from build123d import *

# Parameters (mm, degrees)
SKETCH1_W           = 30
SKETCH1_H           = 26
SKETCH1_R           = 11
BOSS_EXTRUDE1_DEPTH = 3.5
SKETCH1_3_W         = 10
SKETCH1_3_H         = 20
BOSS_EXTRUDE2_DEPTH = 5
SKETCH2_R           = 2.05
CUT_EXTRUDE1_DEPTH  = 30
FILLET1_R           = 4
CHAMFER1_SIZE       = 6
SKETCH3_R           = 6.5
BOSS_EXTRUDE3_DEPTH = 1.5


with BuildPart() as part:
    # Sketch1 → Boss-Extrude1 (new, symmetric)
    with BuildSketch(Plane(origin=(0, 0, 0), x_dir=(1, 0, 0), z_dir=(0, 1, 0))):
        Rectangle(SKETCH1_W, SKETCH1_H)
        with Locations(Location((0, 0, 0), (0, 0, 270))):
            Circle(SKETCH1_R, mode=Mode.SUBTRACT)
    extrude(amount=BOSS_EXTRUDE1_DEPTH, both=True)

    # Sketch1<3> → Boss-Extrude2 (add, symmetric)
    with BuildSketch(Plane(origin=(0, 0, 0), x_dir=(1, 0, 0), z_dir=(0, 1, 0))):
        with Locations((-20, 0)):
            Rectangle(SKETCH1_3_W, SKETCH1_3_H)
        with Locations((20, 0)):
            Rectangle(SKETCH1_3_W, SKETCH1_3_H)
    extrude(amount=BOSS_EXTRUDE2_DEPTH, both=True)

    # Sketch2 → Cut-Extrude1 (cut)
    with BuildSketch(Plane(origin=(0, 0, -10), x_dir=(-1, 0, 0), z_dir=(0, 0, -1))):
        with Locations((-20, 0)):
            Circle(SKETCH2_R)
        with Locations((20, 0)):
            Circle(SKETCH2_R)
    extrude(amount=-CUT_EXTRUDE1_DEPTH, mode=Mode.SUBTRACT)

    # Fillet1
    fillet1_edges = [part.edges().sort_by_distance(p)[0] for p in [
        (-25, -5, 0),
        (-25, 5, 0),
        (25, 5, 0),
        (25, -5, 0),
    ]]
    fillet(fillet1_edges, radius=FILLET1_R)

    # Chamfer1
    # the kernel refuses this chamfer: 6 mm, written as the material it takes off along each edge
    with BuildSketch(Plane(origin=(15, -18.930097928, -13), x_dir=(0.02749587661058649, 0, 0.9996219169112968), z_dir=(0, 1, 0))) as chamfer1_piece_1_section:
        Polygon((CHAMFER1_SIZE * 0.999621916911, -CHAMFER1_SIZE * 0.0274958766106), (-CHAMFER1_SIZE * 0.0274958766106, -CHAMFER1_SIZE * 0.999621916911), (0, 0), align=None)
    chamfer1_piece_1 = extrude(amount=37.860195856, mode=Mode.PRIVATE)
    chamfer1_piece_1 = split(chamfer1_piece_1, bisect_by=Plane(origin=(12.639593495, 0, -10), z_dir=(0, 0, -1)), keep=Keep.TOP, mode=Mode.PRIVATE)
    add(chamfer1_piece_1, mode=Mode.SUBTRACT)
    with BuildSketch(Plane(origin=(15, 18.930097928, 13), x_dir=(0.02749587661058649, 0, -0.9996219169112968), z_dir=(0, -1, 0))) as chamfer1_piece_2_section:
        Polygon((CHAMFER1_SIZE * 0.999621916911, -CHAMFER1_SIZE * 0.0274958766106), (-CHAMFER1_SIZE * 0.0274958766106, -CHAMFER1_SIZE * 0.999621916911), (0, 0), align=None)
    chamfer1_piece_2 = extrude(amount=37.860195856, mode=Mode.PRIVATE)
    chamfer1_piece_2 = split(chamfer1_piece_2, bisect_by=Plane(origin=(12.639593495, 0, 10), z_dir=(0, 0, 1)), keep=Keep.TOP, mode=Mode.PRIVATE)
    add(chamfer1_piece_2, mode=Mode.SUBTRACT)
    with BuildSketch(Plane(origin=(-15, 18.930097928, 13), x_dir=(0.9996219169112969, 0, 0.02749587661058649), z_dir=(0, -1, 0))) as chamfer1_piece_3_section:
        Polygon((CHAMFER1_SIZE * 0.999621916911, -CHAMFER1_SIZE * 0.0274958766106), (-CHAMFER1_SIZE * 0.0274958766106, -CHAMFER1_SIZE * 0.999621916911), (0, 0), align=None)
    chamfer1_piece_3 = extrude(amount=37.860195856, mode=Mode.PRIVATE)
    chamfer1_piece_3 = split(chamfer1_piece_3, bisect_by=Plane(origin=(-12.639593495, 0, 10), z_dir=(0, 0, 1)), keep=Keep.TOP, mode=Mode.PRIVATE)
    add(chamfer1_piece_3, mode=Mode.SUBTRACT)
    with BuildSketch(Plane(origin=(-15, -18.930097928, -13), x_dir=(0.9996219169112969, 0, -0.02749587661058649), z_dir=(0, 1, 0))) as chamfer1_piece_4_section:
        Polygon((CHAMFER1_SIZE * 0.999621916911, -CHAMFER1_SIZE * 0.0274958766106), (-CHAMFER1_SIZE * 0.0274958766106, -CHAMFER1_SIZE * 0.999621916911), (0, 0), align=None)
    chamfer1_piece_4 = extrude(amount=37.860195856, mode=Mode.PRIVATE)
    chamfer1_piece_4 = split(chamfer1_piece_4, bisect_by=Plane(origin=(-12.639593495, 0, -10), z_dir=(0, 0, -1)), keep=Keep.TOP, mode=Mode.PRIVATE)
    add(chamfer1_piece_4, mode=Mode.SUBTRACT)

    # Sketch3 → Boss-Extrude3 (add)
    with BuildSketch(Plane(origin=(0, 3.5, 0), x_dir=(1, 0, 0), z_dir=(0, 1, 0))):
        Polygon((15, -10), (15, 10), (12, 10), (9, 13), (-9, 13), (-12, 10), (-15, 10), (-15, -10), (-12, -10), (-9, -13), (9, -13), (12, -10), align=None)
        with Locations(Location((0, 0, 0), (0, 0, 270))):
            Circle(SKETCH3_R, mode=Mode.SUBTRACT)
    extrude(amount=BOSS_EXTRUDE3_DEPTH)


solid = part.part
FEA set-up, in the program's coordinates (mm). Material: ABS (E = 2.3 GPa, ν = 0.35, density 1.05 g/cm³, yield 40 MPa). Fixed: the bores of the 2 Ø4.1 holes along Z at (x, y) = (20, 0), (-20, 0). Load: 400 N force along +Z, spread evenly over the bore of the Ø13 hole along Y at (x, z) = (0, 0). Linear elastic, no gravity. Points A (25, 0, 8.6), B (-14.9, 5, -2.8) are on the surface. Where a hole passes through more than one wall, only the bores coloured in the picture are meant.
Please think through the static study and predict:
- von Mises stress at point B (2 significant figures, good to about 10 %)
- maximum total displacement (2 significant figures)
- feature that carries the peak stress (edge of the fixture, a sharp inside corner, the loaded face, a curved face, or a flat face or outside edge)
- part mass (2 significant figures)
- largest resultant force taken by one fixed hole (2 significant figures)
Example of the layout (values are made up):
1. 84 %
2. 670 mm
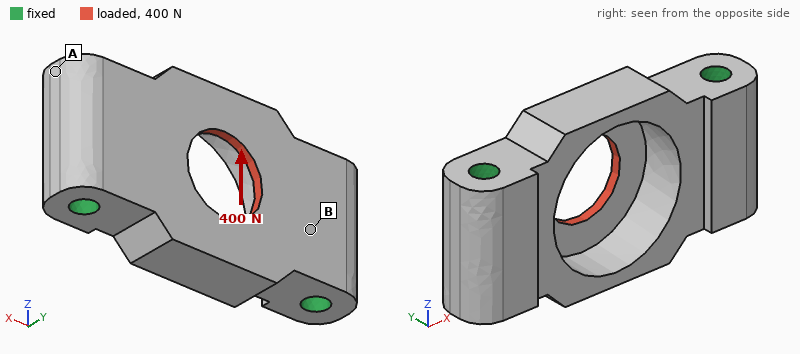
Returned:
1. 3.9 MPa
2. 93 µm
3. a sharp inside corner
4. 6.8 g
5. 200 N
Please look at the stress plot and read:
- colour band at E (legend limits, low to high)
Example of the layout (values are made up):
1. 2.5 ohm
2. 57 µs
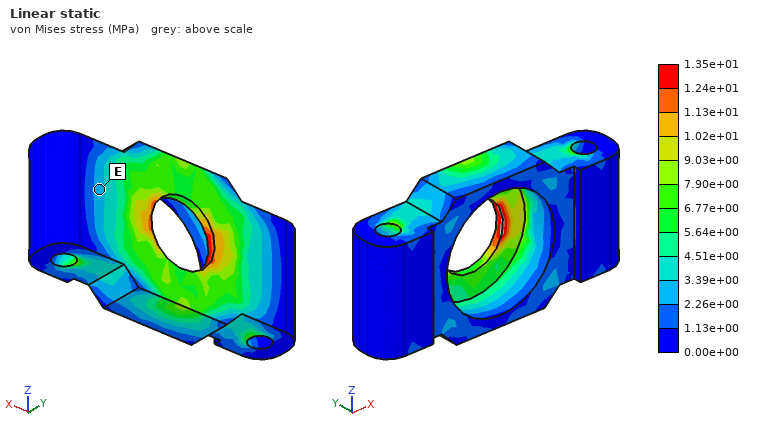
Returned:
1. 2.26e+00 to 3.39e+00 MPa
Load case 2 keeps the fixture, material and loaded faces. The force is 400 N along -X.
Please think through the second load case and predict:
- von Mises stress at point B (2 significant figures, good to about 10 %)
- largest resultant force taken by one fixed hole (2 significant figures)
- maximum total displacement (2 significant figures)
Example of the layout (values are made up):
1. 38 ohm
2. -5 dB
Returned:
1. 3.1 MPa
2. 200 N
3. 39 µm
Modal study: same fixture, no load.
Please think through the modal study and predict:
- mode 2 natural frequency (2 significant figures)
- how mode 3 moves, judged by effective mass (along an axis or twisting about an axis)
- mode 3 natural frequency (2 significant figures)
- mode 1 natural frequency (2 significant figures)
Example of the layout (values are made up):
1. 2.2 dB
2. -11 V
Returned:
1. 7700 Hz
2. along Z
3. 12 kHz
4. 7400 Hz
